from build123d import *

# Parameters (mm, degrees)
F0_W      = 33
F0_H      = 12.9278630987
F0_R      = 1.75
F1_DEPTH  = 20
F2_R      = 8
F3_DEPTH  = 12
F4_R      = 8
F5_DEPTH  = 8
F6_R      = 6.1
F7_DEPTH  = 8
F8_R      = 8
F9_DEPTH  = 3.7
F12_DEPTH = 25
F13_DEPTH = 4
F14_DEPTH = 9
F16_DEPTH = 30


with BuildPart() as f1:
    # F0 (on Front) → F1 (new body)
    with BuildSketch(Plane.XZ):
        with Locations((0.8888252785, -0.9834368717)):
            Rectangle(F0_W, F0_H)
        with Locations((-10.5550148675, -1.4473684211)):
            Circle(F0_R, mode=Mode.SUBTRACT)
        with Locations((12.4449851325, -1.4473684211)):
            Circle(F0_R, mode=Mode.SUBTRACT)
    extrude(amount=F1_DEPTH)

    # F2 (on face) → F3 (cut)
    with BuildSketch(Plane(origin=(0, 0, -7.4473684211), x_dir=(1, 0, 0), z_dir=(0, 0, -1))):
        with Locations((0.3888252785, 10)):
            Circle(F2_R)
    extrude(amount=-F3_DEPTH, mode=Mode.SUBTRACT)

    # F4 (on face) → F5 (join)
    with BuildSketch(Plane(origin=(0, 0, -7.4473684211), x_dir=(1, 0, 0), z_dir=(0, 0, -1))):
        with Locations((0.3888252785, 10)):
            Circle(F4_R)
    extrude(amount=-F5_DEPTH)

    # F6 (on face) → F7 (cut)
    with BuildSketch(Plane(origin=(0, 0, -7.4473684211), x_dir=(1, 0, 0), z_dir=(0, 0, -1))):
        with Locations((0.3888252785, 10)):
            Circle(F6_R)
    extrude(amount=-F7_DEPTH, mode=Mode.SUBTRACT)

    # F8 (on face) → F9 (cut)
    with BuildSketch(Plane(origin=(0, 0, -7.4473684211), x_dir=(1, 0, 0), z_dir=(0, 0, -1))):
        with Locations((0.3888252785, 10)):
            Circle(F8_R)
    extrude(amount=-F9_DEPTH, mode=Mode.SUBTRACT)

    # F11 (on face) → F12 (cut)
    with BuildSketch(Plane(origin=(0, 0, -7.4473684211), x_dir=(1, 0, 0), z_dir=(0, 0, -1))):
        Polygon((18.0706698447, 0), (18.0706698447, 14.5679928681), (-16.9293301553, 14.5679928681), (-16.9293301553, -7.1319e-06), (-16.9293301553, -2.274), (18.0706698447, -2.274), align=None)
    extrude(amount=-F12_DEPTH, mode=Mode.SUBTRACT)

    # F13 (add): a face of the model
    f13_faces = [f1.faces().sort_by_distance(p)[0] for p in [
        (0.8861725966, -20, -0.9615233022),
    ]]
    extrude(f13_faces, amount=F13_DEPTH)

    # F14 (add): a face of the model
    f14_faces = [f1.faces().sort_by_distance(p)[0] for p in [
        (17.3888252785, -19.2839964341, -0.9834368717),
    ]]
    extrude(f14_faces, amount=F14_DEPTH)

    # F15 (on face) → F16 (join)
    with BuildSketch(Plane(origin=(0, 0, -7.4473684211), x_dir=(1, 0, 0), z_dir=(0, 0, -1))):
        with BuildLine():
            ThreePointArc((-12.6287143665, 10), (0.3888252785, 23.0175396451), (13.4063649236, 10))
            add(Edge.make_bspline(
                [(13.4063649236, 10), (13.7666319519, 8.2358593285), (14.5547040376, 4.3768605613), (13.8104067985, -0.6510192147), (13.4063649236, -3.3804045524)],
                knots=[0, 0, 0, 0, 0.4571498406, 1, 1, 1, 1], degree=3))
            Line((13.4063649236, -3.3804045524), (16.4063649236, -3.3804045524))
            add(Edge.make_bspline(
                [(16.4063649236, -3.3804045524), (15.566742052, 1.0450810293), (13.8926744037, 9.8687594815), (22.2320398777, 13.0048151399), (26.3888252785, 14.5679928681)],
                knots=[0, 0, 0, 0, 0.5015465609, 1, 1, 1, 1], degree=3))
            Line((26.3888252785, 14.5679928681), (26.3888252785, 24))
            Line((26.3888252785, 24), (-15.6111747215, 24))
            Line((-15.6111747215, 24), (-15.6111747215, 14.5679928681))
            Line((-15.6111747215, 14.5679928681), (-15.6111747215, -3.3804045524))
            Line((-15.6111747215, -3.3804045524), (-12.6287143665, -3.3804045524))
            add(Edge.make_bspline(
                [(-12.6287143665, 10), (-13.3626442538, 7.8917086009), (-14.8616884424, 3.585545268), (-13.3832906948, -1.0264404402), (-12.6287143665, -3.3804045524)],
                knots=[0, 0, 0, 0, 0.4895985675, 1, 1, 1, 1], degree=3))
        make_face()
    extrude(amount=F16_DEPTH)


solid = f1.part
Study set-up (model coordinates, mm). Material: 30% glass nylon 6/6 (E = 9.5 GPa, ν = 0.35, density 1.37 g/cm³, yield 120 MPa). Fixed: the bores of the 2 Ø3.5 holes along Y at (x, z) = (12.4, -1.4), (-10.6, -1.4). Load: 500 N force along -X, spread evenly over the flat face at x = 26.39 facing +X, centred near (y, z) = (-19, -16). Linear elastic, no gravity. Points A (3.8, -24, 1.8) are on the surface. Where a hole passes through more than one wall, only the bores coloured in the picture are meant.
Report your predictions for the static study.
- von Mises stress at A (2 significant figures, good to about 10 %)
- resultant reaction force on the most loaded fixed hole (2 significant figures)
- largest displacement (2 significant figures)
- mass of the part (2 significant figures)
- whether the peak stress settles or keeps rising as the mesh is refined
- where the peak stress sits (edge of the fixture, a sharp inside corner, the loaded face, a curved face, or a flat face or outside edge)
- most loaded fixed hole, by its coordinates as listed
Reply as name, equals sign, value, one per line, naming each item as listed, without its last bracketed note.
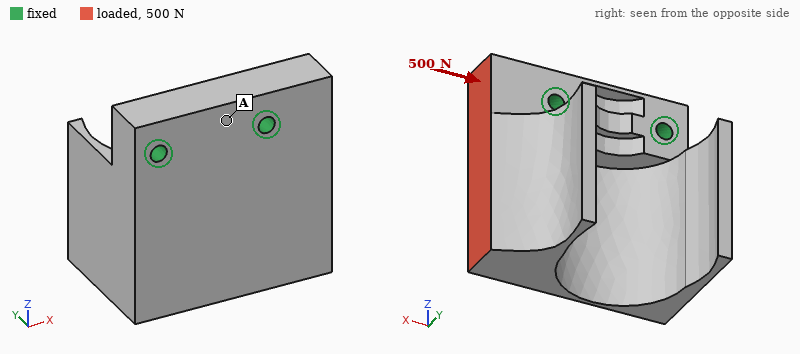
von Mises stress at A = 2.0 MPa
resultant reaction force on the most loaded fixed hole = 450 N
largest displacement = 88 µm
mass of the part = 21 g
whether the peak stress settles or keeps rising as the mesh is refined = keeps rising
where the peak stress sits = edge of the fixture
most loaded fixed hole, by its coordinates as listed = (12.4, -1.4)
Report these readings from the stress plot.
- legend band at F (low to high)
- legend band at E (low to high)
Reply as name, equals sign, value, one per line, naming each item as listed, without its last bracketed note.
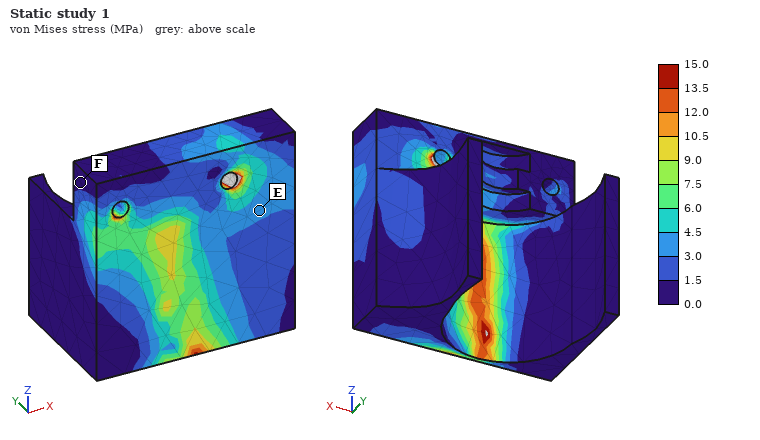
legend band at F = 0.0 to 1.5 MPa
legend band at E = 3.0 to 4.5 MPa
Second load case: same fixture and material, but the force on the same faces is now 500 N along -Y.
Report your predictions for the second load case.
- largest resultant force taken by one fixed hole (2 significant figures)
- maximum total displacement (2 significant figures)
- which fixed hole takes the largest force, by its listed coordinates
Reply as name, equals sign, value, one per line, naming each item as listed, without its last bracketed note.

largest resultant force taken by one fixed hole = 580 N
maximum total displacement = 0.34 mm
which fixed hole takes the largest force, by its listed coordinates = (12.4, -1.4)
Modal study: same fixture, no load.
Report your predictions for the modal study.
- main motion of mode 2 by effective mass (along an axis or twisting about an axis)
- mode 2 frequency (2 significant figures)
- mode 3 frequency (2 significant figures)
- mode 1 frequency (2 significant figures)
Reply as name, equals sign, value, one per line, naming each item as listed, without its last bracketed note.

main motion of mode 2 by effective mass = along Y
mode 2 frequency = 2300 Hz
mode 3 frequency = 2800 Hz
mode 1 frequency = 2200 Hz
